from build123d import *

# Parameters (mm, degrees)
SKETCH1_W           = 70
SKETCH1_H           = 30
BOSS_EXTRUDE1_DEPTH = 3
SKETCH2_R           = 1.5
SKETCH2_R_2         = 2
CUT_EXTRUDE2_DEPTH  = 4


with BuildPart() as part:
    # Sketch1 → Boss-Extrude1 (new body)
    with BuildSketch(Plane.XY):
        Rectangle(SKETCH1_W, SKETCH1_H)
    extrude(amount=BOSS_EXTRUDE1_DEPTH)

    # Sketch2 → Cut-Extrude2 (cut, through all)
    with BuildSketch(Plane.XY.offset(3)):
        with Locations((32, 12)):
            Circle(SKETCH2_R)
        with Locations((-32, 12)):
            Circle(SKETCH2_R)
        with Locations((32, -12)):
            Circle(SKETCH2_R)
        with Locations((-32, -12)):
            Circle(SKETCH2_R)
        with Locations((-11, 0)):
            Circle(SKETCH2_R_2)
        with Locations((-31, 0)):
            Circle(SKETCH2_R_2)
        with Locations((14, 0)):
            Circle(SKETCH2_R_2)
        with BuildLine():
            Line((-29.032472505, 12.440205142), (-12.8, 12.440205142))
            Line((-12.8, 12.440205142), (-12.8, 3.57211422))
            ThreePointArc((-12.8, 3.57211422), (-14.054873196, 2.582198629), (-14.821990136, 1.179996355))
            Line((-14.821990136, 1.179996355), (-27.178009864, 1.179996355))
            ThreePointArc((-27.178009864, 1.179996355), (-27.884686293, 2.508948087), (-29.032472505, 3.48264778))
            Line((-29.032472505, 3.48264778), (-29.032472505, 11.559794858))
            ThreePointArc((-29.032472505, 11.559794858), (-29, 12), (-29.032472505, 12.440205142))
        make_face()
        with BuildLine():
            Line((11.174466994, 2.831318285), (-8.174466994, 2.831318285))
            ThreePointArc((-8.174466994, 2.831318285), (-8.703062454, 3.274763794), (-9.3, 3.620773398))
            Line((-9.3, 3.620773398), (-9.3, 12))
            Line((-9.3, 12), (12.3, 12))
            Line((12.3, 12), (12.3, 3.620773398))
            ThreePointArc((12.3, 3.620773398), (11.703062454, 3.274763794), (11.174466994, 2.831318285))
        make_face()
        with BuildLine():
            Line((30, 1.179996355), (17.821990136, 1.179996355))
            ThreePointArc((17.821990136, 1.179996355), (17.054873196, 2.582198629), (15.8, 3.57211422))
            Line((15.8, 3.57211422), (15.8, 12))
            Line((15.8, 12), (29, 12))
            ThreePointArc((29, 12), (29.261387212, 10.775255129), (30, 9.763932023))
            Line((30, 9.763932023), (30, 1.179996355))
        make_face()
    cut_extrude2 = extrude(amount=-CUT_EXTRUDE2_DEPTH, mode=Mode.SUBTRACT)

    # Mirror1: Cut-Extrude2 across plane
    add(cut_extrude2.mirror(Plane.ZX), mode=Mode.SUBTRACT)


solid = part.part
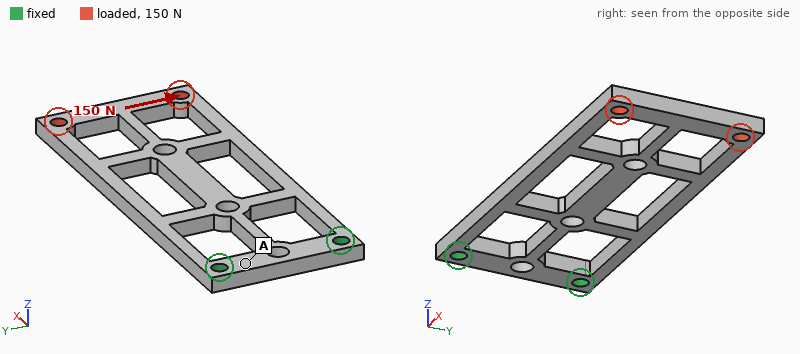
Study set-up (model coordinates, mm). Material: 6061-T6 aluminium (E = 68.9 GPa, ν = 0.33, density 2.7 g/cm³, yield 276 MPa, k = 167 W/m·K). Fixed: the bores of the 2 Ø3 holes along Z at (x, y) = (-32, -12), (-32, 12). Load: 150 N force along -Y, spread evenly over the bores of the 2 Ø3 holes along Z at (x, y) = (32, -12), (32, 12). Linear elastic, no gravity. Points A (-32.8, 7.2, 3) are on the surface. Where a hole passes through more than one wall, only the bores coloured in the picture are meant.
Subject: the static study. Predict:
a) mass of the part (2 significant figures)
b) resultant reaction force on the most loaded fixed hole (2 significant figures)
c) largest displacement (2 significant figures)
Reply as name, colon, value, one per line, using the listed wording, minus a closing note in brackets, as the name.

mass of the part: 8.0 g
resultant reaction force on the most loaded fixed hole: 350 N
largest displacement: 0.33 mm
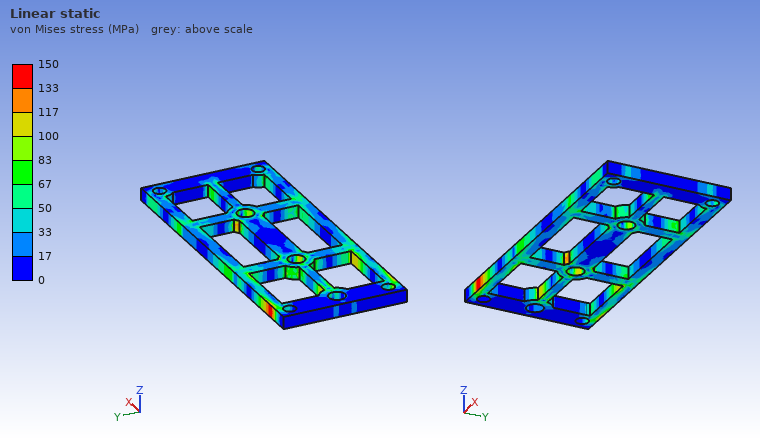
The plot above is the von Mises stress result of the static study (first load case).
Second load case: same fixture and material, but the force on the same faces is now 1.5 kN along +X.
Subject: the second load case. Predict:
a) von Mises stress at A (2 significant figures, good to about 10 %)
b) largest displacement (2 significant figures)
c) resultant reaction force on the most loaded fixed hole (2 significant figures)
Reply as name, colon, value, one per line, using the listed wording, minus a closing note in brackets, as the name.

von Mises stress at A: 27 MPa
largest displacement: 67 µm
resultant reaction force on the most loaded fixed hole: 750 N
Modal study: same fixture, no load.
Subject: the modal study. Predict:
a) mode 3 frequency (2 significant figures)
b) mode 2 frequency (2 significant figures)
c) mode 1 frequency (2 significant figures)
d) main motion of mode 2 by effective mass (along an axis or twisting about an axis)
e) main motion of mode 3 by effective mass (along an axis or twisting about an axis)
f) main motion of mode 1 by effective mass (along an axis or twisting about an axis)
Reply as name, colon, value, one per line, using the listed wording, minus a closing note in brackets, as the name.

mode 3 frequency: 1900 Hz
mode 2 frequency: 1700 Hz
mode 1 frequency: 400 Hz
main motion of mode 2 by effective mass: twisting about X
main motion of mode 3 by effective mass: along Y
main motion of mode 1 by effective mass: along Z
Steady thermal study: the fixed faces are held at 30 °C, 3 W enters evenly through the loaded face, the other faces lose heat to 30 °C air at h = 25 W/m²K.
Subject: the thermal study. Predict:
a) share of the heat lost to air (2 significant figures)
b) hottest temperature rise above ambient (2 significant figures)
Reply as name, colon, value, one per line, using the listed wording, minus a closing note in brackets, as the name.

share of the heat lost to air: 41 %
hottest temperature rise above ambient: 30 K
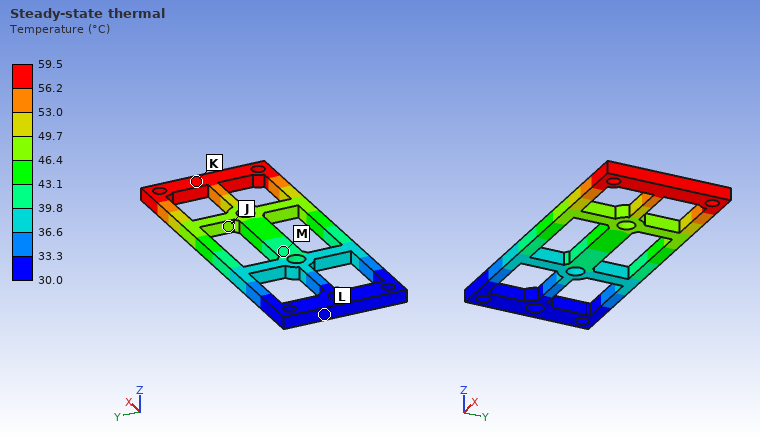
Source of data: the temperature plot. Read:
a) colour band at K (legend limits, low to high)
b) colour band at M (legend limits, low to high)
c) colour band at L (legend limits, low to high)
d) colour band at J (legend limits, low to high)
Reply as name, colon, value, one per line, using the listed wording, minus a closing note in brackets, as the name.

colour band at K: 56.2 to 59.5 °C
colour band at M: 39.8 to 43.1 °C
colour band at L: 30.0 to 33.3 °C
colour band at J: 46.4 to 49.7 °C
